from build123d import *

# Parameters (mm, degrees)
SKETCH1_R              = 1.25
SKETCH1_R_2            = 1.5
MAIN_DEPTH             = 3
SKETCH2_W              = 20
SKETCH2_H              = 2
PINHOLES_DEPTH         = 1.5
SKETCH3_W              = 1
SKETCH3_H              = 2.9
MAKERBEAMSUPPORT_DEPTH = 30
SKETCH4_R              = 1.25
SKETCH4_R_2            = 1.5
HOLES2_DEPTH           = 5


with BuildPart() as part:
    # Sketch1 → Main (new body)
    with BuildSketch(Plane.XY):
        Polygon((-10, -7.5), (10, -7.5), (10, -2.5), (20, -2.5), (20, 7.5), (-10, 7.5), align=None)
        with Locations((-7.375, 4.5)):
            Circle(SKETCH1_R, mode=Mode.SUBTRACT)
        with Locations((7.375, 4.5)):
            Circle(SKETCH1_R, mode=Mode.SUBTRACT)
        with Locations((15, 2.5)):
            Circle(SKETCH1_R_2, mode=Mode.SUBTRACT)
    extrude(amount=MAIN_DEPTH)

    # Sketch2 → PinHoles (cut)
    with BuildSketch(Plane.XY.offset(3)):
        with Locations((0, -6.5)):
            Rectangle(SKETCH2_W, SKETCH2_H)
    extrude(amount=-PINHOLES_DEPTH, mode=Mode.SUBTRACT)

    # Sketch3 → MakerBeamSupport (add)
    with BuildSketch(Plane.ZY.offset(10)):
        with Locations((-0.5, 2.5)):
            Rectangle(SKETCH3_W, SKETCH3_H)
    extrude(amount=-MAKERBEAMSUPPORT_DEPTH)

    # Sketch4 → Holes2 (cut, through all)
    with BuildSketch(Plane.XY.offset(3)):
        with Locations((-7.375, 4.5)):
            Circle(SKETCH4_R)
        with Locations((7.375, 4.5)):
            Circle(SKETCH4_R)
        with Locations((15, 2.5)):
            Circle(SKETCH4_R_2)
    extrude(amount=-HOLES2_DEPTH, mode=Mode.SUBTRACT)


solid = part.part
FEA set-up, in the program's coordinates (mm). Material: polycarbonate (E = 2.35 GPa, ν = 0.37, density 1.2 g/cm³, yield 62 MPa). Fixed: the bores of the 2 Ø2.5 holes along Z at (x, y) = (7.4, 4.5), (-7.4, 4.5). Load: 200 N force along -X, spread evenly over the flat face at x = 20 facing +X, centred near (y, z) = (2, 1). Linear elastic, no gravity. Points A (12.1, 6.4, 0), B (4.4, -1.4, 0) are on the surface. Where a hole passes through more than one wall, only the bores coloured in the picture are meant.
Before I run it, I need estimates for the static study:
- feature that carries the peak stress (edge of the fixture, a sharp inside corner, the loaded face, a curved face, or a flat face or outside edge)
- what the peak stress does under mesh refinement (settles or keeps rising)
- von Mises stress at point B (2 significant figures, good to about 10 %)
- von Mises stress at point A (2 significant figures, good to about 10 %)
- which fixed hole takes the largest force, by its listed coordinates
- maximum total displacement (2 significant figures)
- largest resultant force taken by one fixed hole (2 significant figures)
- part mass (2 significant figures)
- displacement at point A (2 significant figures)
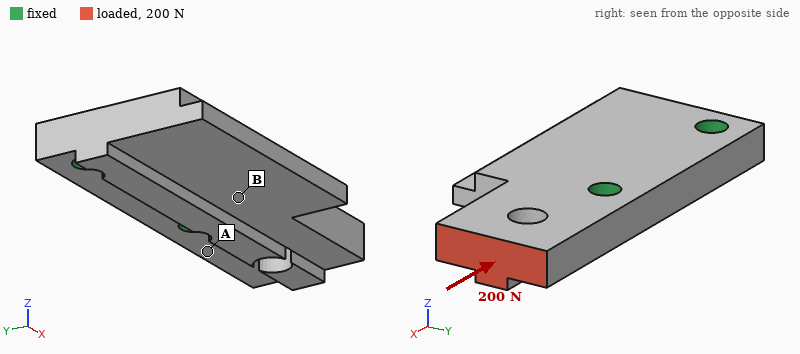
a sharp inside corner
keeps rising
2.8 MPa
9.3 MPa
(7.4, 4.5)
78 µm
170 N
1.4 g
15 µm
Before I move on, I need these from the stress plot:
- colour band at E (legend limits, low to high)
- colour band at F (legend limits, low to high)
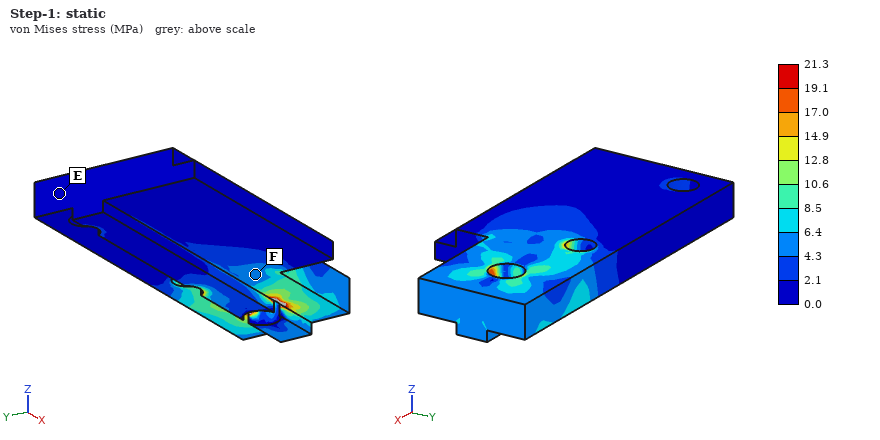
0.0 to 2.1 MPa
4.3 to 6.4 MPa
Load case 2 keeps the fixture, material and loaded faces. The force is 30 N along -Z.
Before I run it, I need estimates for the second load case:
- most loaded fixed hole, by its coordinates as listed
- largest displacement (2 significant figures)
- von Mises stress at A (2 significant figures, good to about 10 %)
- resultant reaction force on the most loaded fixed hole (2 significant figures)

(7.4, 4.5)
0.34 mm
14 MPa
36 N
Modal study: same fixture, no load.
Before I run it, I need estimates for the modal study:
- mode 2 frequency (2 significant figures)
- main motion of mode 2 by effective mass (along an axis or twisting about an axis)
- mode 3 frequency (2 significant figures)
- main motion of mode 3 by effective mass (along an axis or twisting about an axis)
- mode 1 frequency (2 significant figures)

6000 Hz
along Z
8300 Hz
along Y
4600 Hz
